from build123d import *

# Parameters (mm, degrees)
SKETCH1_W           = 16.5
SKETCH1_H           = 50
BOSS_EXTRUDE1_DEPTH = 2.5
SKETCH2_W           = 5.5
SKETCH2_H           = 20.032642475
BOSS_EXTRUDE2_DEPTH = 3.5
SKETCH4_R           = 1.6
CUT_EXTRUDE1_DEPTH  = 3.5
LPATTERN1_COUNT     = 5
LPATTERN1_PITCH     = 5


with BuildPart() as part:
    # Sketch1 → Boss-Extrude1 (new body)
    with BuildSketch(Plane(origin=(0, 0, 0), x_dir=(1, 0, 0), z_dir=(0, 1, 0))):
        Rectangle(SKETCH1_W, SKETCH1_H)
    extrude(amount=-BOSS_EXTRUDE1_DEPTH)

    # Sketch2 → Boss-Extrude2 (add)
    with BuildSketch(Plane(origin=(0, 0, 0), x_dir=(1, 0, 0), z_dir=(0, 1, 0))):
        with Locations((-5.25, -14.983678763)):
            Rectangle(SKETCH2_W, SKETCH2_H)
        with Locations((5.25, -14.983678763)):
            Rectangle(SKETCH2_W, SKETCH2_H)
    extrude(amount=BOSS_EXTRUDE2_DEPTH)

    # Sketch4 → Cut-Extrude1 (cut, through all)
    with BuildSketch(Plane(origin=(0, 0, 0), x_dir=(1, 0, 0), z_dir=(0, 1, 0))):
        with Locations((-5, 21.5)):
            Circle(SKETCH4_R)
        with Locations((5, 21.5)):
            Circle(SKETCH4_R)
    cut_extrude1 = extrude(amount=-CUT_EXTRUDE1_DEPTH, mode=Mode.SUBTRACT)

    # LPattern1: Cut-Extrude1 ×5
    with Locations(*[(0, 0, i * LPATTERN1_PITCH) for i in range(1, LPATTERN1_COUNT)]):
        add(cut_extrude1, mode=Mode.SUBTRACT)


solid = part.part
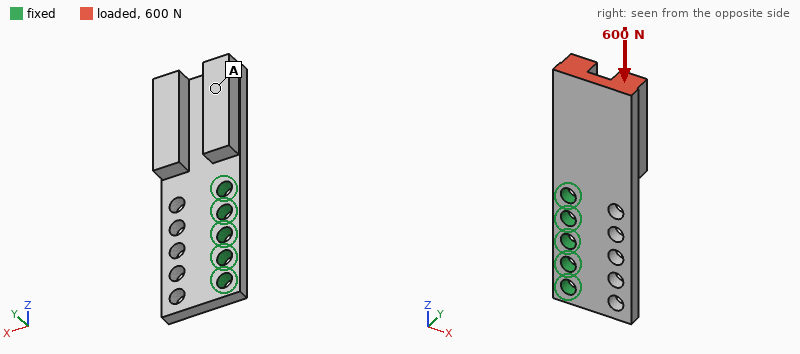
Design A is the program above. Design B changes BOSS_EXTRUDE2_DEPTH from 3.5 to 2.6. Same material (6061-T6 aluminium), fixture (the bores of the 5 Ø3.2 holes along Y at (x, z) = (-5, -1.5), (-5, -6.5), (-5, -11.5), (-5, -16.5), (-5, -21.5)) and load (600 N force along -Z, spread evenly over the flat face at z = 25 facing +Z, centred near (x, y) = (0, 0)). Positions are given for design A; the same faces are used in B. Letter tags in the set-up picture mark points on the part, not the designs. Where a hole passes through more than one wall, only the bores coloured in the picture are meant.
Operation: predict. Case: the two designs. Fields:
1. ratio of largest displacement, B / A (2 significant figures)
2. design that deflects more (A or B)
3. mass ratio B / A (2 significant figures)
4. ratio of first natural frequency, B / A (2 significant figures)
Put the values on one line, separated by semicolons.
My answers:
0.72; A; 0.92; 1.1
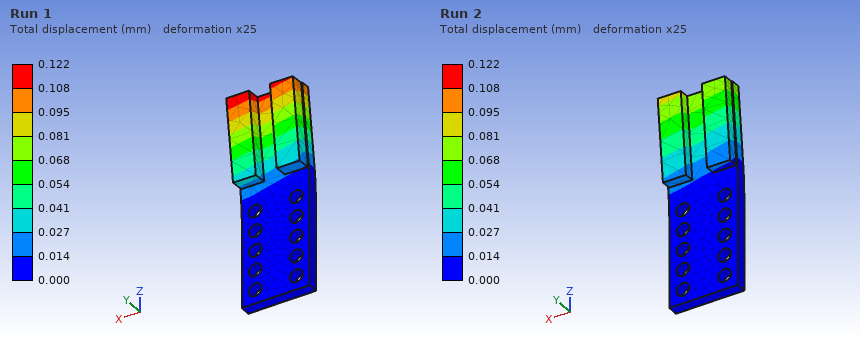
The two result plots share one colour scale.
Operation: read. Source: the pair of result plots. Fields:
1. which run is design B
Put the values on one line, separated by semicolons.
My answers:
Run 2
